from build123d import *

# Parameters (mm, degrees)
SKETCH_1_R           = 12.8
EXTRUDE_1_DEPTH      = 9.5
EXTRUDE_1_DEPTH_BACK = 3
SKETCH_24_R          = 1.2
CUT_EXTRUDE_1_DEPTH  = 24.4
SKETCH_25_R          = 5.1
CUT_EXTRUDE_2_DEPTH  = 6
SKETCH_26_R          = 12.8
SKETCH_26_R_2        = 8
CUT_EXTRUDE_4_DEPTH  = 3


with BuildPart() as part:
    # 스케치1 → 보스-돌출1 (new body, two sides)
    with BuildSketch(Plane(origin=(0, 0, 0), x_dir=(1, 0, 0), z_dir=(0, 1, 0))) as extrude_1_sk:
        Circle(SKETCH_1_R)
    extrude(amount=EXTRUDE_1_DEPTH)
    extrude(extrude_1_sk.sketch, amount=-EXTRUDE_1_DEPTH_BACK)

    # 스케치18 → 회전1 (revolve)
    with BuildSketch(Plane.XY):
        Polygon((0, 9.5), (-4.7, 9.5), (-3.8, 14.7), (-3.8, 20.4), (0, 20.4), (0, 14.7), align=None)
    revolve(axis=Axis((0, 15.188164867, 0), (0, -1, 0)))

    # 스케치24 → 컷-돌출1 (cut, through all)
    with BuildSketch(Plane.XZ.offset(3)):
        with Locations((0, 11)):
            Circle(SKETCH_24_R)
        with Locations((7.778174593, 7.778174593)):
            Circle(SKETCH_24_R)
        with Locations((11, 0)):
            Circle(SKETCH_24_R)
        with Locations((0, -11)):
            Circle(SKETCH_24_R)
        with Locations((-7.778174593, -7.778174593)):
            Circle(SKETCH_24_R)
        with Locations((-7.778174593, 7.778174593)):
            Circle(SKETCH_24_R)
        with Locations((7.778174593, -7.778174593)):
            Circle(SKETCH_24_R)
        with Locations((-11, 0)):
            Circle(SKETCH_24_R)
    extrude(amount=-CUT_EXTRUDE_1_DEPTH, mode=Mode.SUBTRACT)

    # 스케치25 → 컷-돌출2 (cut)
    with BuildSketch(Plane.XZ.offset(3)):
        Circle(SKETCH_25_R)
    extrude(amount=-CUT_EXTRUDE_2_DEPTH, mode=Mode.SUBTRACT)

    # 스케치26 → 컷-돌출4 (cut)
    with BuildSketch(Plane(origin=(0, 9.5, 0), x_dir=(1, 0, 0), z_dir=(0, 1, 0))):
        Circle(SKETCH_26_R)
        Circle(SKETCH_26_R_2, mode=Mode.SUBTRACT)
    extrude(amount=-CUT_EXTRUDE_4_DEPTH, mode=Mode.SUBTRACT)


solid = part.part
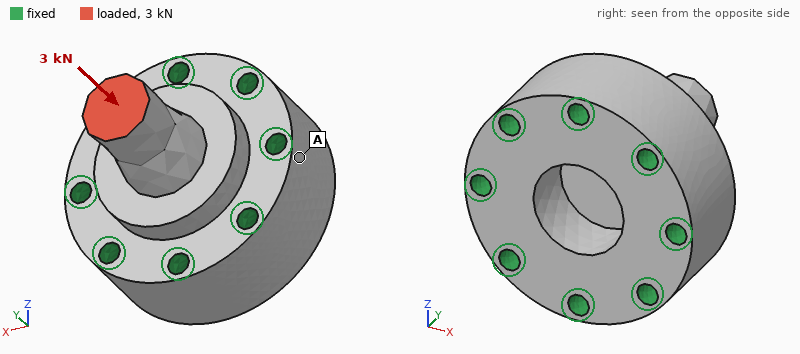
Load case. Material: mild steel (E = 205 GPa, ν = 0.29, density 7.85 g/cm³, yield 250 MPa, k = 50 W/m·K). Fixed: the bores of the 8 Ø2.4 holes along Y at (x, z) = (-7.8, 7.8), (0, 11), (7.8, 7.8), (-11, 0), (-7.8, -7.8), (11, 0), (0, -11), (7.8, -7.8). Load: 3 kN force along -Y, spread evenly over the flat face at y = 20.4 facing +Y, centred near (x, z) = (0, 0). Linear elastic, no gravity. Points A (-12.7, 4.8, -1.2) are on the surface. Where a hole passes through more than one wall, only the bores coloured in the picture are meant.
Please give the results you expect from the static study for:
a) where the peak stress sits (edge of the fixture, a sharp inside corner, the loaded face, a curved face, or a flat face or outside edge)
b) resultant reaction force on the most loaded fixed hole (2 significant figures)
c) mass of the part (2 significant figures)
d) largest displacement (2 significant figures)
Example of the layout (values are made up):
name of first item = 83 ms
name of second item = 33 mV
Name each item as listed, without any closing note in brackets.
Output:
where the peak stress sits = a sharp inside corner
resultant reaction force on the most loaded fixed hole = 460 N
mass of the part = 41 g
largest displacement = 4.5 µm
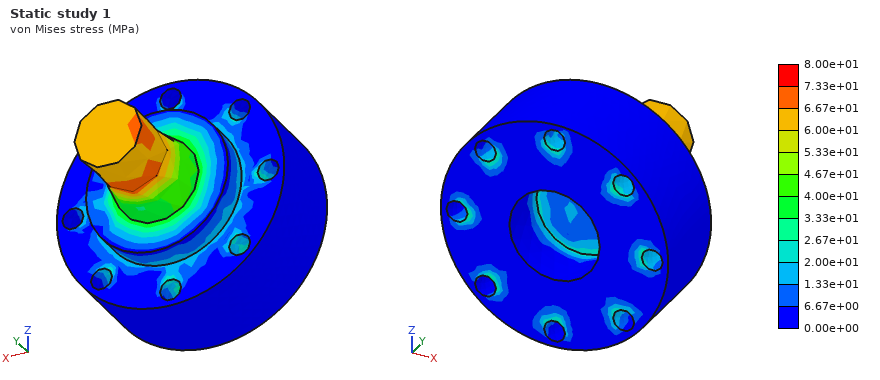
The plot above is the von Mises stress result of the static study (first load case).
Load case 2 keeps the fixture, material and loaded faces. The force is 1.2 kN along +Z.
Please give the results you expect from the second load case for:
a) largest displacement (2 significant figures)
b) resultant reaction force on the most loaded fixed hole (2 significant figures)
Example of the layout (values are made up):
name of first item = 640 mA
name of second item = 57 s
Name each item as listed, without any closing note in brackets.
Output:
largest displacement = 21 µm
resultant reaction force on the most loaded fixed hole = 630 N
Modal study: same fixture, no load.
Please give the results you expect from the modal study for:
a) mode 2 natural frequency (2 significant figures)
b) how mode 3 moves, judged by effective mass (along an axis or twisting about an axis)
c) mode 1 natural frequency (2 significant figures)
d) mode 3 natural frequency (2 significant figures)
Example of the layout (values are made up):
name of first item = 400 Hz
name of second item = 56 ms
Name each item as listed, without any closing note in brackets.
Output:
mode 2 natural frequency = 36 kHz
how mode 3 moves, judged by effective mass = along Y
mode 1 natural frequency = 36 kHz
mode 3 natural frequency = 73 kHz
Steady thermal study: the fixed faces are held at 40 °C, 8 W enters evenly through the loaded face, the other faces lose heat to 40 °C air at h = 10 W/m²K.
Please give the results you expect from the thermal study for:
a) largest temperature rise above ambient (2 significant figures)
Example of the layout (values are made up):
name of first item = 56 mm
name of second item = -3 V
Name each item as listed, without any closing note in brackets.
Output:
largest temperature rise above ambient = 43 K
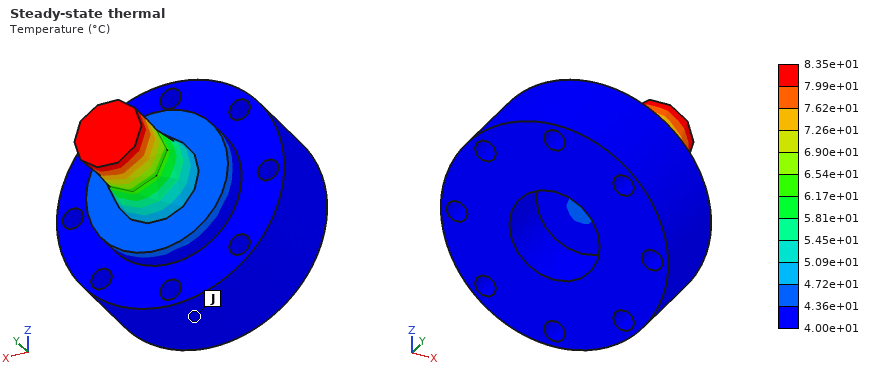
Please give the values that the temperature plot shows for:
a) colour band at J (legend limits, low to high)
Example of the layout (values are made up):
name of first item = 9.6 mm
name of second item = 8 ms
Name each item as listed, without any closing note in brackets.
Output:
colour band at J = 4.00e+01 to 4.36e+01 °C
